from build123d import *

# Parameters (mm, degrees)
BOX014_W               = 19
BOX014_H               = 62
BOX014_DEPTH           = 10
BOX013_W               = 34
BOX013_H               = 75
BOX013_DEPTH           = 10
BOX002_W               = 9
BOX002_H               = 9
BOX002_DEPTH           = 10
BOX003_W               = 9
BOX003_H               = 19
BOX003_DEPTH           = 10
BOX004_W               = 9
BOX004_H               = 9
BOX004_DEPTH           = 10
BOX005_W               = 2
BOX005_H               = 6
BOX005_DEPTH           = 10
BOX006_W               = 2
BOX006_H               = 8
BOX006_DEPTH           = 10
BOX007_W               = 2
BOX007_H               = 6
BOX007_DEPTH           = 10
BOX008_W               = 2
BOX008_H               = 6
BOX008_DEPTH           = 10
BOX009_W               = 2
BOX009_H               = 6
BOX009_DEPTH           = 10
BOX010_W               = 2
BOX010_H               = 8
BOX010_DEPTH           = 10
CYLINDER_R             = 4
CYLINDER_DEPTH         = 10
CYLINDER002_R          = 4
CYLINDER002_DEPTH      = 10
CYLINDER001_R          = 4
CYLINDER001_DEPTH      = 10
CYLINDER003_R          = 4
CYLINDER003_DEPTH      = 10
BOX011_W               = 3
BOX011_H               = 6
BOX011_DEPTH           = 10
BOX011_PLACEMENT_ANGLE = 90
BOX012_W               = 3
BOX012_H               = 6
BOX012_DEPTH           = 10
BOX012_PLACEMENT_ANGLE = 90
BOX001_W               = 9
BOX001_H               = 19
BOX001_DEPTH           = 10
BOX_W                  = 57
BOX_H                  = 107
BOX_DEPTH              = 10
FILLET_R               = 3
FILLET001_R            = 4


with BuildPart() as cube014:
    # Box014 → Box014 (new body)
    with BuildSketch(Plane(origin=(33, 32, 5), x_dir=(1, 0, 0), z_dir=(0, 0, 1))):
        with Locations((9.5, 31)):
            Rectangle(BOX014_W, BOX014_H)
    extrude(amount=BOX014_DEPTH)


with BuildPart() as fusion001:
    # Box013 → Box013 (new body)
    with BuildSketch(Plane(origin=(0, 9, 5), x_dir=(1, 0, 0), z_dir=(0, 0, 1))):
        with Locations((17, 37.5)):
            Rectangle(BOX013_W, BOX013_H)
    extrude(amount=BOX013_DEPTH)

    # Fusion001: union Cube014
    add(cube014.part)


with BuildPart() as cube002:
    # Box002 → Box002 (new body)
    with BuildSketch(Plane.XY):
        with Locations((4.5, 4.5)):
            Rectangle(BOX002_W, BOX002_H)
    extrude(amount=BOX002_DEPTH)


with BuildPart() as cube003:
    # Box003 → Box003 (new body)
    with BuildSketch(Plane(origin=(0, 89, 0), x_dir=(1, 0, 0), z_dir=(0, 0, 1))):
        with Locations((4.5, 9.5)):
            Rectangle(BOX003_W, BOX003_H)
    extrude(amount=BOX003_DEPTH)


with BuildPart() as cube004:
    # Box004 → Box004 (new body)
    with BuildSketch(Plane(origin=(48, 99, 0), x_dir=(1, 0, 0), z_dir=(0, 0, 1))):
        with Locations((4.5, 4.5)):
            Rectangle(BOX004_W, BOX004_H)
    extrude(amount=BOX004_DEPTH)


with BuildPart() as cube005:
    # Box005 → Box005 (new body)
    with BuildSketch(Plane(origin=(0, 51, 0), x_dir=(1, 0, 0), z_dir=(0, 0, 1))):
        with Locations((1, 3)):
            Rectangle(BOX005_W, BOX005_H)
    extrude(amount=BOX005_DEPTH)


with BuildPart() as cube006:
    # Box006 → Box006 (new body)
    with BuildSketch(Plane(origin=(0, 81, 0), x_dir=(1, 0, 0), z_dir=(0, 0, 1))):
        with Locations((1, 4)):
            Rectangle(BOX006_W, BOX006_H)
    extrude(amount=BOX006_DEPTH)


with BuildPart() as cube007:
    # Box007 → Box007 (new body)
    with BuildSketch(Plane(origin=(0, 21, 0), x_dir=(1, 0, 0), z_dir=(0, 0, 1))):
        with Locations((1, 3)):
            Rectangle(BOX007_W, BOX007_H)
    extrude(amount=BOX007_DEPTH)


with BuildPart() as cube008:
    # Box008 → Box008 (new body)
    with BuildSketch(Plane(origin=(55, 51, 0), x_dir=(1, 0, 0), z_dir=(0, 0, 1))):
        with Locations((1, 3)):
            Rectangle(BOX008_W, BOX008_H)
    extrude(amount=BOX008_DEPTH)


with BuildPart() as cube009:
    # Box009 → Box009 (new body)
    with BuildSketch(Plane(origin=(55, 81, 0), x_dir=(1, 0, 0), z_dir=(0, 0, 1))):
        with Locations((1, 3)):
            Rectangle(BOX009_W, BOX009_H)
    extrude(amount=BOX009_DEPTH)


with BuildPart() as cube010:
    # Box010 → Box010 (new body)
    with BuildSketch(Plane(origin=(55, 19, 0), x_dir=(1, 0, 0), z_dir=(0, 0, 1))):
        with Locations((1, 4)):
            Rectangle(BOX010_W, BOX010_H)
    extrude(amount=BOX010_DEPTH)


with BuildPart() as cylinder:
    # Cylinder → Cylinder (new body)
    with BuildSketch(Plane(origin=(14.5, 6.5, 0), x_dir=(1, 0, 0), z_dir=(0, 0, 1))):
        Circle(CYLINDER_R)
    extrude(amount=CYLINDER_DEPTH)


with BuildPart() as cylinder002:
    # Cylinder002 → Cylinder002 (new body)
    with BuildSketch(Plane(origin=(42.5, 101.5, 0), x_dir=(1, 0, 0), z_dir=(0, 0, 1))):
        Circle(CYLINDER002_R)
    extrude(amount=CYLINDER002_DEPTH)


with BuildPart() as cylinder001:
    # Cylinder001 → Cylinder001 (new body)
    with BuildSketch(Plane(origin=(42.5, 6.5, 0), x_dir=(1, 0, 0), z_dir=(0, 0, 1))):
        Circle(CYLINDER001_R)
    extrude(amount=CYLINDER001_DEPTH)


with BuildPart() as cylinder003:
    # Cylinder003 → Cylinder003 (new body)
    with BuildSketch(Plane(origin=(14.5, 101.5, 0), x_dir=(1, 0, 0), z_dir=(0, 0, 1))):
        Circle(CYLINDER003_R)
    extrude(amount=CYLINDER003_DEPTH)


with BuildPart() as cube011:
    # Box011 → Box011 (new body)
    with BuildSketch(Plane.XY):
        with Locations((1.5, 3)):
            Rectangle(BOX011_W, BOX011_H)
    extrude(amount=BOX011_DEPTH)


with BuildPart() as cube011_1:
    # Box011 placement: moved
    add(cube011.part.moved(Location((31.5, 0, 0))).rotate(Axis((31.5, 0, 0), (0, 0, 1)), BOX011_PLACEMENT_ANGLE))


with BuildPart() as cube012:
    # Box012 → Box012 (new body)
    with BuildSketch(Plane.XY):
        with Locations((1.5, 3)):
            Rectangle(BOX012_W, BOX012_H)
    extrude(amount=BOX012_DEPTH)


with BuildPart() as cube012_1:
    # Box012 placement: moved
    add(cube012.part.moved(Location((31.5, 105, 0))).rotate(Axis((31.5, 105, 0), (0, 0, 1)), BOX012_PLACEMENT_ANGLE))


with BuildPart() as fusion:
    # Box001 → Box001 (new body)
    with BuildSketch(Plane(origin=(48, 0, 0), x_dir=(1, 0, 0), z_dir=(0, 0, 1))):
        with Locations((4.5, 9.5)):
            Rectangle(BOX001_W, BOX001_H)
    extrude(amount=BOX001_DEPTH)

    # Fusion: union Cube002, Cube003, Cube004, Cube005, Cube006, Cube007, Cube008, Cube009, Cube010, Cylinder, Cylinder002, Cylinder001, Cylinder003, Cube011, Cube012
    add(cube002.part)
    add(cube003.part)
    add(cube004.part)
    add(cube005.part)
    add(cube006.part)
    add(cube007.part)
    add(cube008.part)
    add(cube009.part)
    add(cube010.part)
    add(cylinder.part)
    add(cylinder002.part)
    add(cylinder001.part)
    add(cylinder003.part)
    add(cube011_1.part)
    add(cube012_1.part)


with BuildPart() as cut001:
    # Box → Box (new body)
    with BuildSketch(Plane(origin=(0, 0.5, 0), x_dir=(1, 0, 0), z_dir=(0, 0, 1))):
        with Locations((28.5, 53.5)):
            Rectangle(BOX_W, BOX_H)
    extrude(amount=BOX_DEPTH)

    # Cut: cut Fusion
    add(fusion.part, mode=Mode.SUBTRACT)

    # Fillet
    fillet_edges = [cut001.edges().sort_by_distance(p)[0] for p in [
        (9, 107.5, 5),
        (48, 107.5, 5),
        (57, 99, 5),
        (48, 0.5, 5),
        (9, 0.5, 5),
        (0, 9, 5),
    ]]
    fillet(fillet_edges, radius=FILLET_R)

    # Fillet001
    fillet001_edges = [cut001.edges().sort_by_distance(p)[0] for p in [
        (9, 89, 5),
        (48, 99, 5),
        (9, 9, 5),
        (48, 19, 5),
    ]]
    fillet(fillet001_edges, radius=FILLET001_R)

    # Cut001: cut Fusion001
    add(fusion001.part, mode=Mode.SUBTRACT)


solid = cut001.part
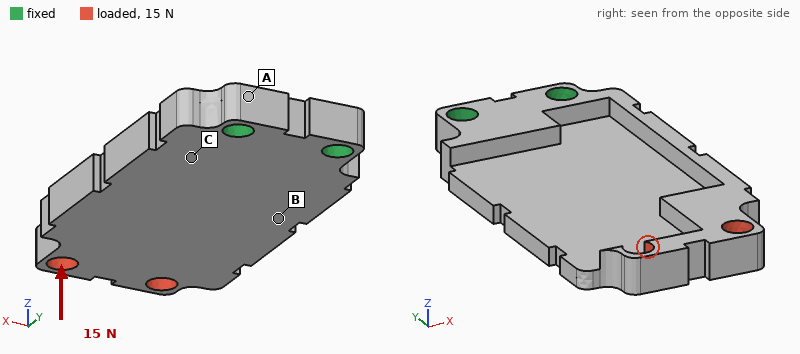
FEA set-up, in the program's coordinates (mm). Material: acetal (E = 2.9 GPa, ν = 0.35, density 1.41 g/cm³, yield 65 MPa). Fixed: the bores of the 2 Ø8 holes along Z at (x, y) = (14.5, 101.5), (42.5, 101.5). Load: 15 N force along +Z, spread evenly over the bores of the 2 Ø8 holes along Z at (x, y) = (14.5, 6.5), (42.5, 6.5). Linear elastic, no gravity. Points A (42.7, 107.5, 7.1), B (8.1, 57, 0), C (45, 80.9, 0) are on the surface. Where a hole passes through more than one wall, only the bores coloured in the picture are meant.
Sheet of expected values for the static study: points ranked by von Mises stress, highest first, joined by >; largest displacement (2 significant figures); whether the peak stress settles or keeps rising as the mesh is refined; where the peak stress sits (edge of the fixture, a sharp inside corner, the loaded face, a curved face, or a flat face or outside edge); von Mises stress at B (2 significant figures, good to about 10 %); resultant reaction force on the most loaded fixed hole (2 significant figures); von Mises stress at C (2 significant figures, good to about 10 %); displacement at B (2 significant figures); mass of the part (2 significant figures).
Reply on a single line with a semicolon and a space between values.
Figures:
C > B > A; 1.3 mm; keeps rising; a sharp inside corner; 2.1 MPa; 14 N; 3.1 MPa; 0.25 mm; 49 g
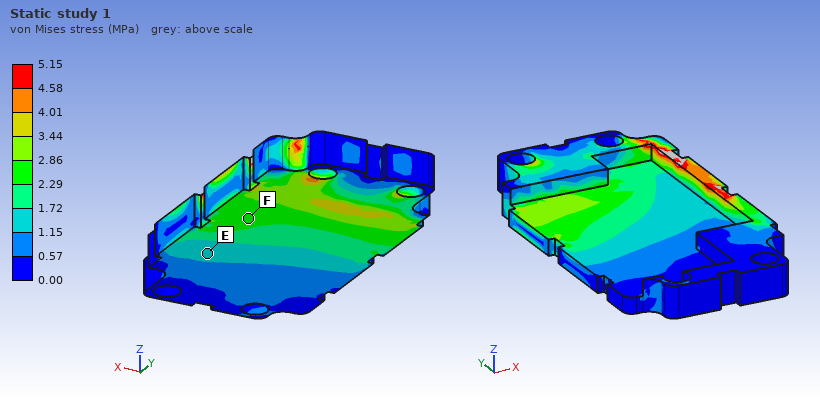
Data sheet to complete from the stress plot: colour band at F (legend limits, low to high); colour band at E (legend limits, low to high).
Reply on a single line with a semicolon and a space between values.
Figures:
2.29 to 2.86 MPa; 1.15 to 1.72 MPa
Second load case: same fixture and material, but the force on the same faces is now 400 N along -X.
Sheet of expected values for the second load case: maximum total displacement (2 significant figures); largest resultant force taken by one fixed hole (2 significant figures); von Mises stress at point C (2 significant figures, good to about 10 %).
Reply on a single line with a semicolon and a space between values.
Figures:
1.4 mm; 1.2 kN; 9.7 MPa
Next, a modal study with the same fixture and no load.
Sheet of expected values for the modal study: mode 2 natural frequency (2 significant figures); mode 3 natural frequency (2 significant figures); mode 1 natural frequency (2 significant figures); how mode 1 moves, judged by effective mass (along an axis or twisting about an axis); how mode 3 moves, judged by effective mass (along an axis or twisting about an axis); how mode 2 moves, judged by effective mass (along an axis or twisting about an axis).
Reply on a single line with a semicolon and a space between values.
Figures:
530 Hz; 900 Hz; 160 Hz; along Z; along X; twisting about Y
